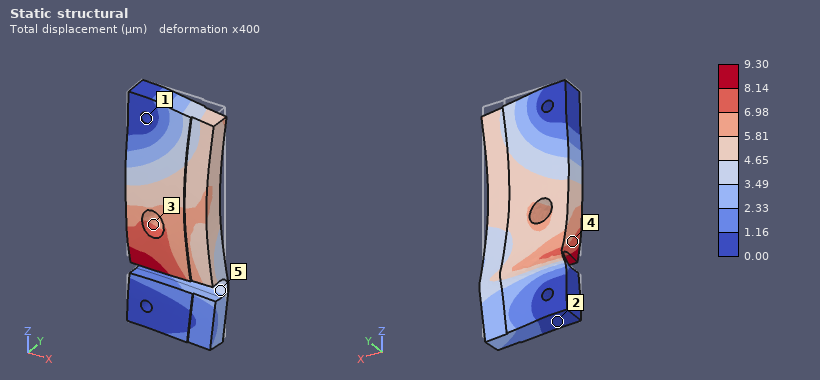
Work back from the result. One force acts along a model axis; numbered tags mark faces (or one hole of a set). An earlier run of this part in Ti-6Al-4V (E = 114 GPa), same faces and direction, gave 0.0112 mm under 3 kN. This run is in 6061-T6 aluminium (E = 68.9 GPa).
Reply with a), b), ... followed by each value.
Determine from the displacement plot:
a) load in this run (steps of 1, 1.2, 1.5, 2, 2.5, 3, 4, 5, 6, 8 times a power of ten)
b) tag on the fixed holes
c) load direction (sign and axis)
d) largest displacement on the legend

a) 1.5 kN
b) 1
c) -Z
d) 9.30 µm
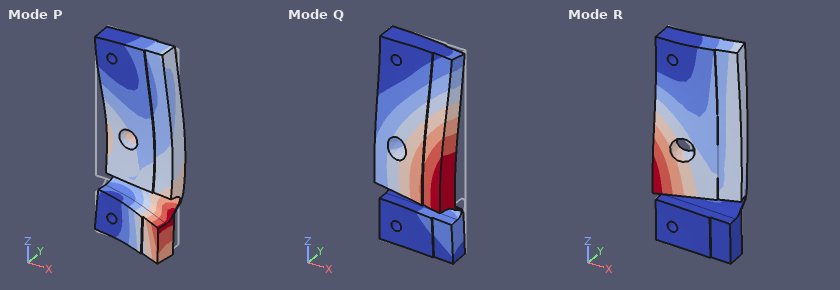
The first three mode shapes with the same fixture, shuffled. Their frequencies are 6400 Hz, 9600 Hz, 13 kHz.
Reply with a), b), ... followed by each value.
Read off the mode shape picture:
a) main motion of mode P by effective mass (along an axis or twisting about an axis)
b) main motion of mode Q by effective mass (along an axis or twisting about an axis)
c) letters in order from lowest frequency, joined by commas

a) along X
b) along Y
c) Q, R, P
